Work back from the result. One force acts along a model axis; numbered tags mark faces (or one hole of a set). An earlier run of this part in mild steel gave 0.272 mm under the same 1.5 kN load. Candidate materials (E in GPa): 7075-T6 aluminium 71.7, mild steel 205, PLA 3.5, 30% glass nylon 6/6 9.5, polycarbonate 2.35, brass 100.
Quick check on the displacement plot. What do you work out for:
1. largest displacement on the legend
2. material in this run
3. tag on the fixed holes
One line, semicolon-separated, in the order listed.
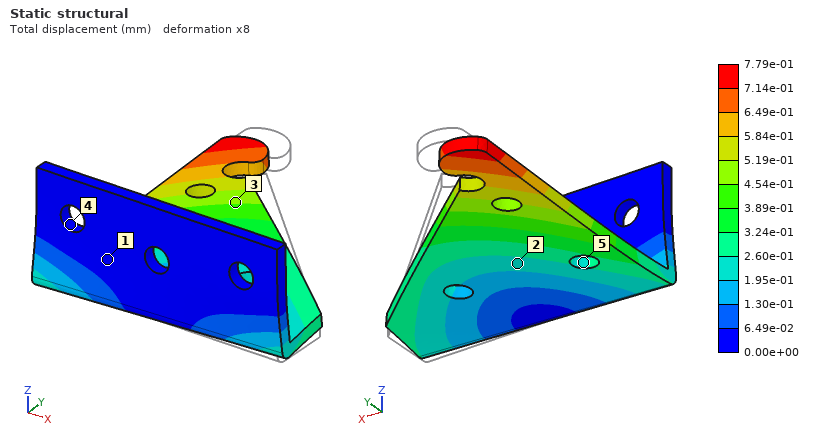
7.79e-01 mm; 7075-T6 aluminium; 4
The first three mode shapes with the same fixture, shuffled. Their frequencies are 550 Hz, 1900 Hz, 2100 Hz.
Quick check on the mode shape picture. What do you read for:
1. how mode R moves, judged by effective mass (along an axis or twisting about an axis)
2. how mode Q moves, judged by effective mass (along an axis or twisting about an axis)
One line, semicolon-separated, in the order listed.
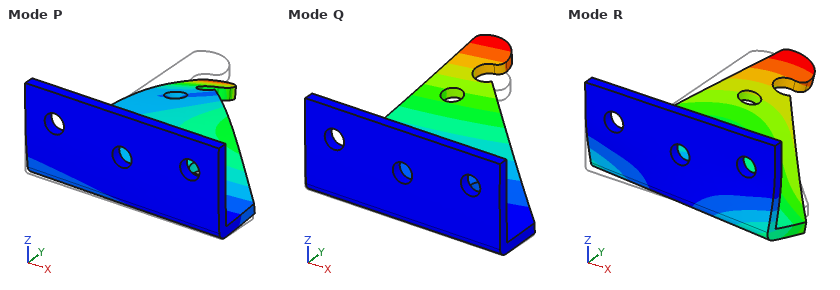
along X; along Z
